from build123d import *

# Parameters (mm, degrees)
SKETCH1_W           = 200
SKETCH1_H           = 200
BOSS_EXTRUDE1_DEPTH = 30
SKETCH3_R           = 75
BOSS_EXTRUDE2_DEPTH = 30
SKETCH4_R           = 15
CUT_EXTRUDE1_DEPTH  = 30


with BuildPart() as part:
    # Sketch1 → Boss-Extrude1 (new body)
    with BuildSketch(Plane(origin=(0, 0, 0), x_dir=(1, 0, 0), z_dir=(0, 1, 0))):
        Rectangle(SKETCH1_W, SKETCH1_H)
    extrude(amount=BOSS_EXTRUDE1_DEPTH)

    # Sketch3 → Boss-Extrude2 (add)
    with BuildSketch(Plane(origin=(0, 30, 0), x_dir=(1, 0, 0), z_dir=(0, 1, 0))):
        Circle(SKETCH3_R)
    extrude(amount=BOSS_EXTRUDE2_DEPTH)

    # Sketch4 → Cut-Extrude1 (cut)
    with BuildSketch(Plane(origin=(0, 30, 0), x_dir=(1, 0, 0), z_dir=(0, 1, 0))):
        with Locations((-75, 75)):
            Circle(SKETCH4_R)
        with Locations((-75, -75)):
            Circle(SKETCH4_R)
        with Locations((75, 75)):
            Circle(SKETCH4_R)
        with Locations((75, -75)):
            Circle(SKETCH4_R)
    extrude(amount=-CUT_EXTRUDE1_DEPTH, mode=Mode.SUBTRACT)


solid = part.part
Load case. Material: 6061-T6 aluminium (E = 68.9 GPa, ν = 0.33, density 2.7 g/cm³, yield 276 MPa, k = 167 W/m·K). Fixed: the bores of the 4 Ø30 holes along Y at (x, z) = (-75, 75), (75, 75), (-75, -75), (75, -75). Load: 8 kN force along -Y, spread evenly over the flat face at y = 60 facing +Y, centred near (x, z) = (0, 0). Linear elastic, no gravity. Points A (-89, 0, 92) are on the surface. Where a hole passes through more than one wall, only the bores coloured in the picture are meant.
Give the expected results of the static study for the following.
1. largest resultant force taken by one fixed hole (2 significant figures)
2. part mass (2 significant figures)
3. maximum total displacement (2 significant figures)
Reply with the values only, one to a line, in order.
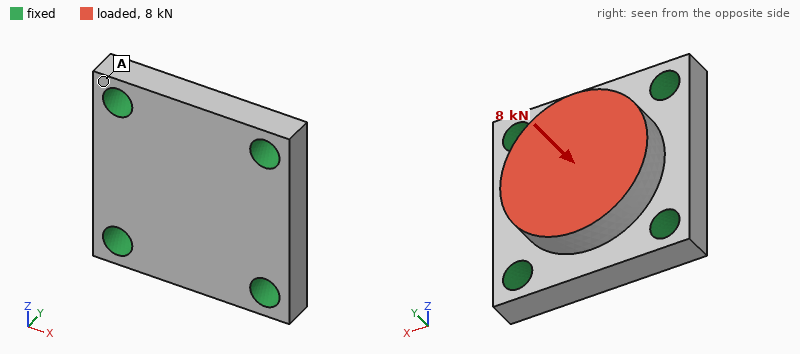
2.1 kN
4.4 kg
2.9 µm
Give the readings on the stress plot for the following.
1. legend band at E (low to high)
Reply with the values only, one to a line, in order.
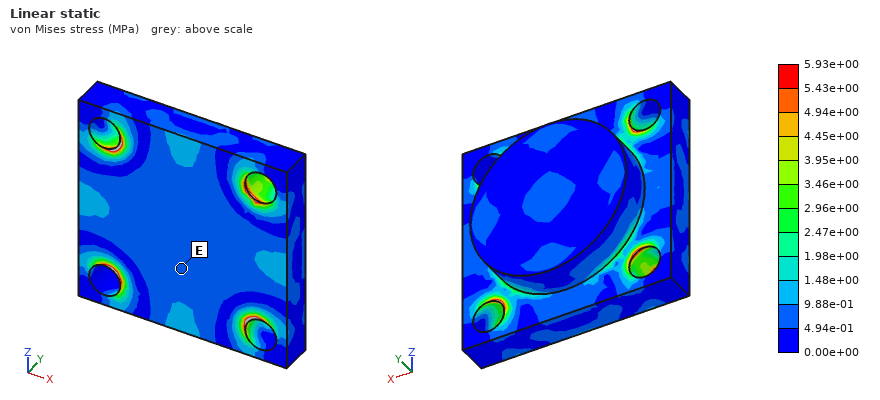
4.94e-01 to 9.88e-01 MPa
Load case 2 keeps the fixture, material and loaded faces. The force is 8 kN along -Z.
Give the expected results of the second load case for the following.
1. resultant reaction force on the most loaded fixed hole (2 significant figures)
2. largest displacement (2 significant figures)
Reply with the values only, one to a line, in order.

2.6 kN
3.4 µm
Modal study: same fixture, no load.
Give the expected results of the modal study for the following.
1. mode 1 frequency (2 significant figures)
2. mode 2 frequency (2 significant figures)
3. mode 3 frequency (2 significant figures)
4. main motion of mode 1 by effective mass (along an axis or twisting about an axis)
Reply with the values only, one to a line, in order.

5000 Hz
6700 Hz
6700 Hz
along Y
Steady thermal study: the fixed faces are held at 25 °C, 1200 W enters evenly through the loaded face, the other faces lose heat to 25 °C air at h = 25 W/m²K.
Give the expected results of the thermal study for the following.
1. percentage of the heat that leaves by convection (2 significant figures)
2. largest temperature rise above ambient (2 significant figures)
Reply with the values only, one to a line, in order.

3.4 %
45 K
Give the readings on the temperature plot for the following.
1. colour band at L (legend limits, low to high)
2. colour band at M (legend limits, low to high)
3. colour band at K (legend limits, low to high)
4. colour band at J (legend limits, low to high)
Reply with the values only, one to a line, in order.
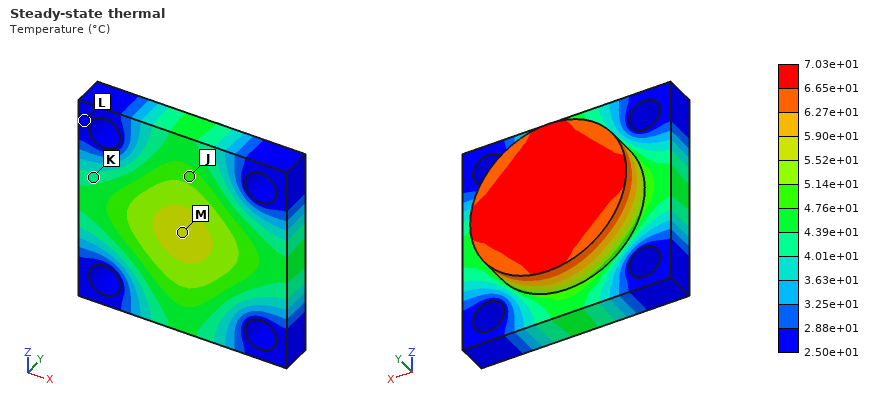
2.50e+01 to 2.88e+01 °C
5.52e+01 to 5.90e+01 °C
4.01e+01 to 4.39e+01 °C
4.76e+01 to 5.14e+01 °C
